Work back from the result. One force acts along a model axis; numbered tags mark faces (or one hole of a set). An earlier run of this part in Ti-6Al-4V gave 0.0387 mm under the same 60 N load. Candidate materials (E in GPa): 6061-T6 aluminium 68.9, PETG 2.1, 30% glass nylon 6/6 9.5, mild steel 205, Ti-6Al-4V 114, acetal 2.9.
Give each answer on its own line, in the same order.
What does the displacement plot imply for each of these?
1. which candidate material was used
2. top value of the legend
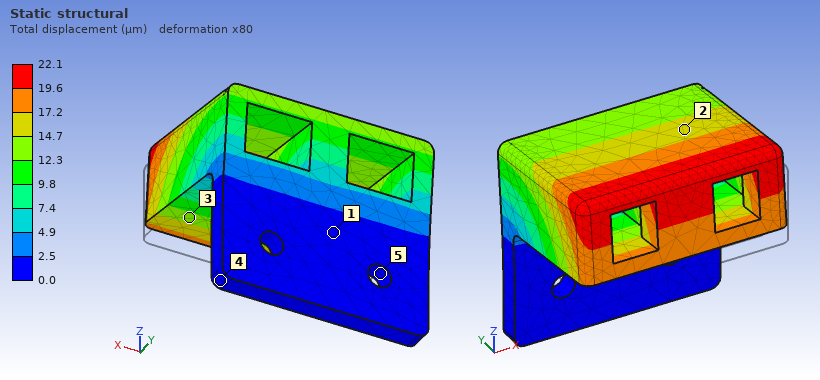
mild steel
22.1 µm
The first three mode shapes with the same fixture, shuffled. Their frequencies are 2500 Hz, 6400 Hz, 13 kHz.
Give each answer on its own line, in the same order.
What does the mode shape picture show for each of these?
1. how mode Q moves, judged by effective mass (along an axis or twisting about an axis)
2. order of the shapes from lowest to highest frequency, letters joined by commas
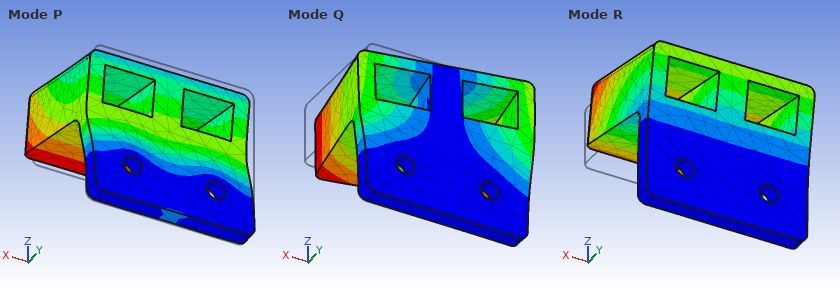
along X
R, Q, P
